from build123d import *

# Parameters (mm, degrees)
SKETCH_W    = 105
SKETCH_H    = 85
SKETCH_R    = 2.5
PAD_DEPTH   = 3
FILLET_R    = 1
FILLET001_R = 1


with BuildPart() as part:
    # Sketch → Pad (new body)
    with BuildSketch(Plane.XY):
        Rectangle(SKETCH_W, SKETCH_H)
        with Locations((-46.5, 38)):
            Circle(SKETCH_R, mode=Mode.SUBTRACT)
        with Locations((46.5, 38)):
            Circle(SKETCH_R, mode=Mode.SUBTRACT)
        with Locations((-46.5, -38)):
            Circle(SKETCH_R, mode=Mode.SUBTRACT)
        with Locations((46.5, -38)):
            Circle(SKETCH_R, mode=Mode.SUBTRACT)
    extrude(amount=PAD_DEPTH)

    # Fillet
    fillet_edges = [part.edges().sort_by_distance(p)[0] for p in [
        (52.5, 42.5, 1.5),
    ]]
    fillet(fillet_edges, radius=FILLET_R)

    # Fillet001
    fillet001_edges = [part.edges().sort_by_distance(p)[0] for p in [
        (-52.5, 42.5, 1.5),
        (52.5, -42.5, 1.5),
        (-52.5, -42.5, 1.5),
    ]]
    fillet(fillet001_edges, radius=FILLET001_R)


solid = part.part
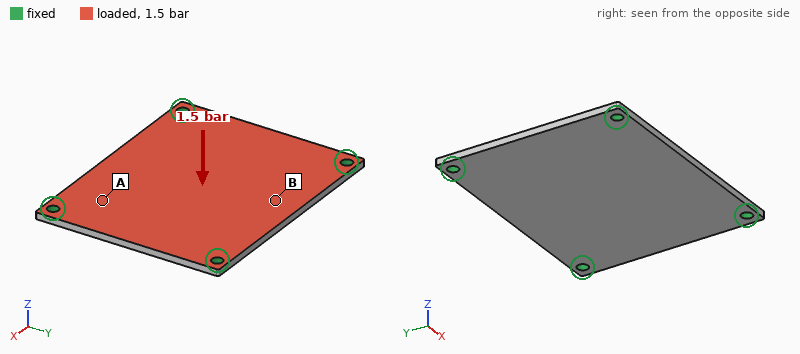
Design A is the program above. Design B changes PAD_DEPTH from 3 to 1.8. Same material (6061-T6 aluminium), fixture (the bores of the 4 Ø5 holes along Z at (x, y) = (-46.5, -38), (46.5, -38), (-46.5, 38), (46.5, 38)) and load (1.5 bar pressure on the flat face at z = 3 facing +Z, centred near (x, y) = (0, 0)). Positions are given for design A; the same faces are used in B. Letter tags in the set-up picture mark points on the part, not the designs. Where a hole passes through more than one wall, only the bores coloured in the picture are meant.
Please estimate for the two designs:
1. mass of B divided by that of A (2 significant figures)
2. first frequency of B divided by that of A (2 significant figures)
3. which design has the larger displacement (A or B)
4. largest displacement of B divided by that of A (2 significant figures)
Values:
0.60
0.61
B
4.4
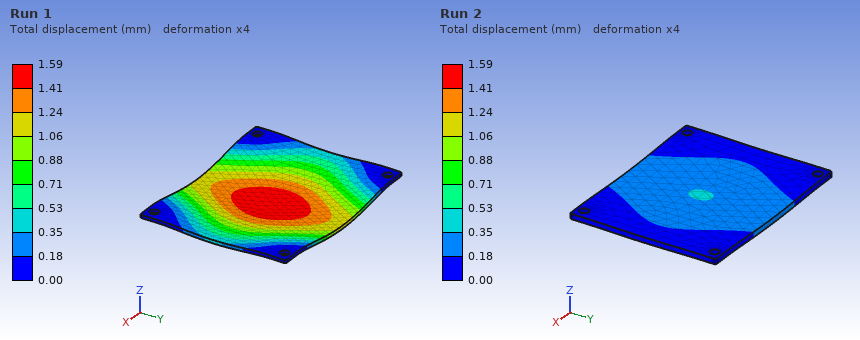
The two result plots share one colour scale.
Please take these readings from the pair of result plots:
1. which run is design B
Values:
Run 1
